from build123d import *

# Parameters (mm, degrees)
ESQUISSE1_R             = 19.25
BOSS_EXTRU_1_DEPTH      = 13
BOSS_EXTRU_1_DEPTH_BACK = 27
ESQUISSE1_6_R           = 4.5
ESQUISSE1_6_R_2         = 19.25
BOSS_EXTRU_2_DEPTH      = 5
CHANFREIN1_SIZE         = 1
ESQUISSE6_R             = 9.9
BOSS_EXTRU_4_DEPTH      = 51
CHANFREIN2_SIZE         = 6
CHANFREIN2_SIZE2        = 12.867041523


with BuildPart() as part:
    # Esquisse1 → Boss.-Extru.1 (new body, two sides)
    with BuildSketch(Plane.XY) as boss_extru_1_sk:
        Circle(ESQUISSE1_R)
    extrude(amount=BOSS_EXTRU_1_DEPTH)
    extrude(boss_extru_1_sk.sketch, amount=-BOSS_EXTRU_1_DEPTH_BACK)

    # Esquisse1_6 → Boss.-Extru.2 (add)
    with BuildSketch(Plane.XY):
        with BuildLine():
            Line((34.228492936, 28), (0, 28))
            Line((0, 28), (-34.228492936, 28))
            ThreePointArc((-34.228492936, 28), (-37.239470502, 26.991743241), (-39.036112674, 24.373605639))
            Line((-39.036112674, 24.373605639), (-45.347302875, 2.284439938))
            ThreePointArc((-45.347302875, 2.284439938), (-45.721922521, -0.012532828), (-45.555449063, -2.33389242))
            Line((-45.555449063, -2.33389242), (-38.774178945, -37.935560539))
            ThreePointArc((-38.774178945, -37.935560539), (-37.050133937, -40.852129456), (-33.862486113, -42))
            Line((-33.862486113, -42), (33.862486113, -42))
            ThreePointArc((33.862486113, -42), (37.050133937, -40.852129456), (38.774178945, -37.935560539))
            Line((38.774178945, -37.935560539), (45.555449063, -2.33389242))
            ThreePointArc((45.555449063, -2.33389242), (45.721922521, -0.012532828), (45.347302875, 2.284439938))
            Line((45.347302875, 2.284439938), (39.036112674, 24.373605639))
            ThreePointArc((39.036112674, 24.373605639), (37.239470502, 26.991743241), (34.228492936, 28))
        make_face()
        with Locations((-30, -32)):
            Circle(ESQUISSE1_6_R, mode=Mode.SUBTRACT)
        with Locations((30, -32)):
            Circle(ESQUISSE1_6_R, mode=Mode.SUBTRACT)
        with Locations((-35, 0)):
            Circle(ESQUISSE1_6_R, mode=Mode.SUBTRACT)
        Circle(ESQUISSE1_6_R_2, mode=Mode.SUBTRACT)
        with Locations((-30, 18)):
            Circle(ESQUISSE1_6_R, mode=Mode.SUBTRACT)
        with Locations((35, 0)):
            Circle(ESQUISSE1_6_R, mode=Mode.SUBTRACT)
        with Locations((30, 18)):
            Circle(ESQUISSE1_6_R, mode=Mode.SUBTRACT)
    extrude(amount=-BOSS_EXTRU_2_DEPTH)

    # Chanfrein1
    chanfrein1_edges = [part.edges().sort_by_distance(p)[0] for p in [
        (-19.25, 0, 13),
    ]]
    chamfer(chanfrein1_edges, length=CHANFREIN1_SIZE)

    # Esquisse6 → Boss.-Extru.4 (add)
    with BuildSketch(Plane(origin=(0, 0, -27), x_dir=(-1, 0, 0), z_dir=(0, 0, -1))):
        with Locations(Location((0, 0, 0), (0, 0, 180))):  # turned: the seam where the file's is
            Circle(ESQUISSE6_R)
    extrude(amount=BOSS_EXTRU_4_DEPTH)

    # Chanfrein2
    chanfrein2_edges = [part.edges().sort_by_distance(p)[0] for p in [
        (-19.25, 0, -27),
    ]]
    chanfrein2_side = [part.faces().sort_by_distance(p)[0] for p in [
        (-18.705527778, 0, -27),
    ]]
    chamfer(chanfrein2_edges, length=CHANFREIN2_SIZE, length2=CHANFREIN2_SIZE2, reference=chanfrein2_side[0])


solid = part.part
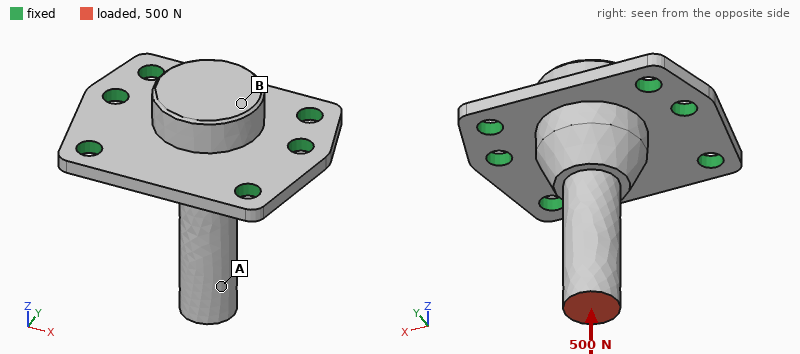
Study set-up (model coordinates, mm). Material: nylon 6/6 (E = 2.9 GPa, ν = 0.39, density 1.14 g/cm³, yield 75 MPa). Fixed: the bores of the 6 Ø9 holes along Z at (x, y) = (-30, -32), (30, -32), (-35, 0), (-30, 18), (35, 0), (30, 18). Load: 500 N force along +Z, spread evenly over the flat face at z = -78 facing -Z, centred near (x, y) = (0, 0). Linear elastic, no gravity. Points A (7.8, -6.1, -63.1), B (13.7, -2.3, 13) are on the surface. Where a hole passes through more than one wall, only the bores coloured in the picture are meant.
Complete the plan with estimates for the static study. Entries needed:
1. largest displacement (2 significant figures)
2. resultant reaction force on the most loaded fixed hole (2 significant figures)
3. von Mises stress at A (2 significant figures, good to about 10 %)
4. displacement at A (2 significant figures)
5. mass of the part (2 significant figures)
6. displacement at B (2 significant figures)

0.11 mm
110 N
1.6 MPa
0.093 mm
91 g
0.060 mm
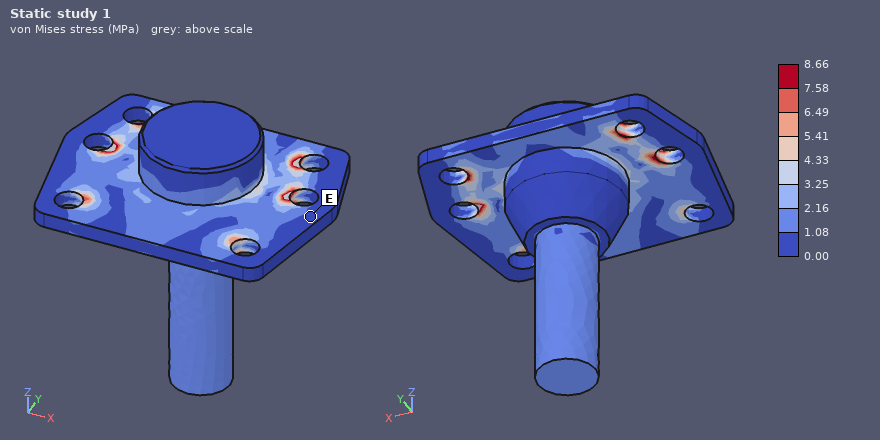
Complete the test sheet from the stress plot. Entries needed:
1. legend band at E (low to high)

0.00 to 1.08 MPa
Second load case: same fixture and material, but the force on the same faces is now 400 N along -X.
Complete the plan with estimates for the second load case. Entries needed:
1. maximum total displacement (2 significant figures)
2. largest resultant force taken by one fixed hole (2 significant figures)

1.7 mm
320 N
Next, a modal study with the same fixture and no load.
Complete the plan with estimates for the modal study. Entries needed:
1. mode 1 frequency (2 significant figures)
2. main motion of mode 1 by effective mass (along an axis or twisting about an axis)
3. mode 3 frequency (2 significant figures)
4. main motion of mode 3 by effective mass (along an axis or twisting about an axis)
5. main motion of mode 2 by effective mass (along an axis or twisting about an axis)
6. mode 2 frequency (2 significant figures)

750 Hz
along Y
1700 Hz
along Z
along X
980 Hz
